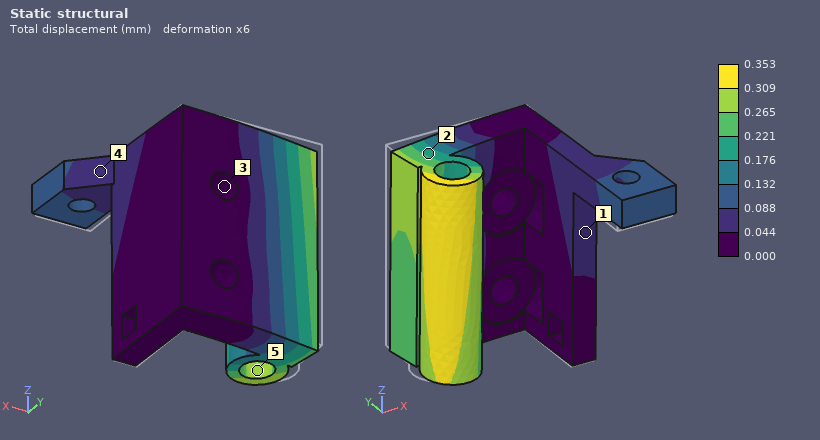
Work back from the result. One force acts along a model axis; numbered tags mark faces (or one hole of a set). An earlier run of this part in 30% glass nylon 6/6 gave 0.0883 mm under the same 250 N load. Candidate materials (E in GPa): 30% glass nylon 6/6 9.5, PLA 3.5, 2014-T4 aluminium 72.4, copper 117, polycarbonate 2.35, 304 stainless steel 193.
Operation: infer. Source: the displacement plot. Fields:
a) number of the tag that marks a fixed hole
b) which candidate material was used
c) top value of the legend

3
polycarbonate
0.353 mm
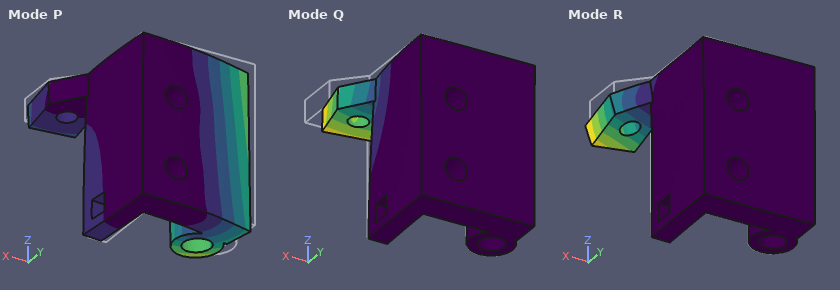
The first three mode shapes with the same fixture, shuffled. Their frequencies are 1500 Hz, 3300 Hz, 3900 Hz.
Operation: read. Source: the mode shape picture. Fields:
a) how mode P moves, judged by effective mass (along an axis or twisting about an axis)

along Y
